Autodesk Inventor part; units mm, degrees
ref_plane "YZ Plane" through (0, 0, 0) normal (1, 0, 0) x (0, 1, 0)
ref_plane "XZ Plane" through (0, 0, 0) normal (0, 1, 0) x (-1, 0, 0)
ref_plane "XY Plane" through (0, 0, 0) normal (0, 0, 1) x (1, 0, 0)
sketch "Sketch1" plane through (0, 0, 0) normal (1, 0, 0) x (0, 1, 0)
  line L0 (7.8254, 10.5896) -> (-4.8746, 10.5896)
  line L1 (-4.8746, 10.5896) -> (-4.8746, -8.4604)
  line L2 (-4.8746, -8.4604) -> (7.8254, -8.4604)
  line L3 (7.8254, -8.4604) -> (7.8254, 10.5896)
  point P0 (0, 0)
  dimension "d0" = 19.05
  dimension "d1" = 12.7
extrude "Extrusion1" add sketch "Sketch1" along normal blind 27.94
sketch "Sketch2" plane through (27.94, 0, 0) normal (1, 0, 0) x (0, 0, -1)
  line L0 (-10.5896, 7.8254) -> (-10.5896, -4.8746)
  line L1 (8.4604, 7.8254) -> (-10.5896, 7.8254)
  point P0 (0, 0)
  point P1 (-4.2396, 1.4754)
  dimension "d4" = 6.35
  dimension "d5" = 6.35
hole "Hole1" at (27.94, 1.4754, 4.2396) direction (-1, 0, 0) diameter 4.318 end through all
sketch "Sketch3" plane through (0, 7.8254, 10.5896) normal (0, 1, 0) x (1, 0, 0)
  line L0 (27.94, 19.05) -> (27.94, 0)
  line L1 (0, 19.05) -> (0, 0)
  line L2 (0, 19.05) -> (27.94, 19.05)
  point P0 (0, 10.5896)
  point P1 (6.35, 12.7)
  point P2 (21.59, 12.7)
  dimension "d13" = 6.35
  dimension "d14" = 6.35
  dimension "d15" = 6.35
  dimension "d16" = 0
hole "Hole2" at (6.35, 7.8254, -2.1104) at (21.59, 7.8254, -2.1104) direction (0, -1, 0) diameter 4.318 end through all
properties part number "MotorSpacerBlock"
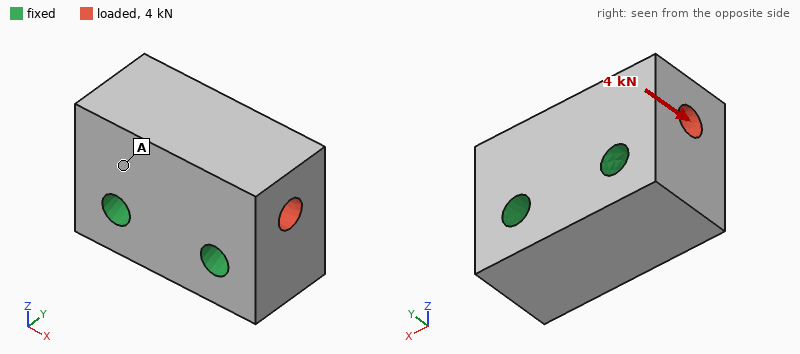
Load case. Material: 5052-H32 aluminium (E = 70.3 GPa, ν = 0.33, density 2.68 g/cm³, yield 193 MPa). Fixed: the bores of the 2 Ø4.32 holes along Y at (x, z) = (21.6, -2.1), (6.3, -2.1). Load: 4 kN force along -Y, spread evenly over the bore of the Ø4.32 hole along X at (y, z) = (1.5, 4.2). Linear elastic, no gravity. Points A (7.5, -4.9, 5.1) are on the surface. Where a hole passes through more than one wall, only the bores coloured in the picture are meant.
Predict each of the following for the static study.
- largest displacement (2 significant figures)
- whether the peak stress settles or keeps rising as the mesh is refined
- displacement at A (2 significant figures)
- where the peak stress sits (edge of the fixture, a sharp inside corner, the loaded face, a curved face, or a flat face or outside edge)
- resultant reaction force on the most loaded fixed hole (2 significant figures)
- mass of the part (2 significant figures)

7.9 µm
keeps rising
5.4 µm
edge of the fixture
2.0 kN
16 g
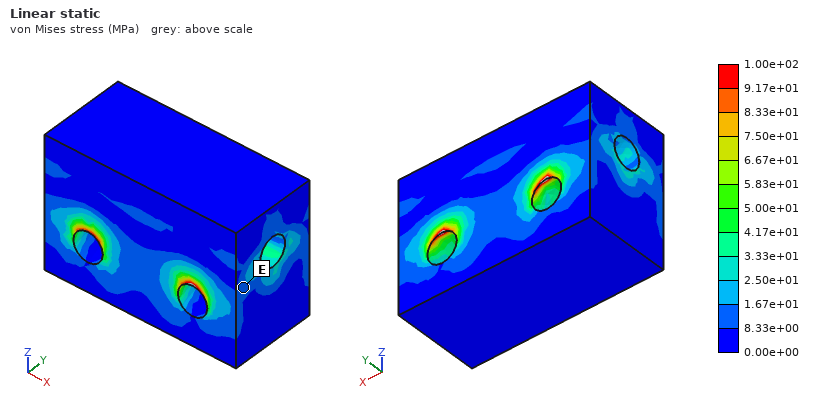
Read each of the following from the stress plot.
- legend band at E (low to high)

8.33e+00 to 1.67e+01 MPa
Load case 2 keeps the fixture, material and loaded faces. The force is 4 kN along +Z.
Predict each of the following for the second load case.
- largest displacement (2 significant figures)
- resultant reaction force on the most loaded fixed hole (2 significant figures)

2.3 µm
2.0 kN
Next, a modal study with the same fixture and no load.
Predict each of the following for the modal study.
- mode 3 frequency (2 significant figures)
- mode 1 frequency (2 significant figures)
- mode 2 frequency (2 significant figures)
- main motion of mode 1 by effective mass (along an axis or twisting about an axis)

49 kHz
38 kHz
48 kHz
along Y
